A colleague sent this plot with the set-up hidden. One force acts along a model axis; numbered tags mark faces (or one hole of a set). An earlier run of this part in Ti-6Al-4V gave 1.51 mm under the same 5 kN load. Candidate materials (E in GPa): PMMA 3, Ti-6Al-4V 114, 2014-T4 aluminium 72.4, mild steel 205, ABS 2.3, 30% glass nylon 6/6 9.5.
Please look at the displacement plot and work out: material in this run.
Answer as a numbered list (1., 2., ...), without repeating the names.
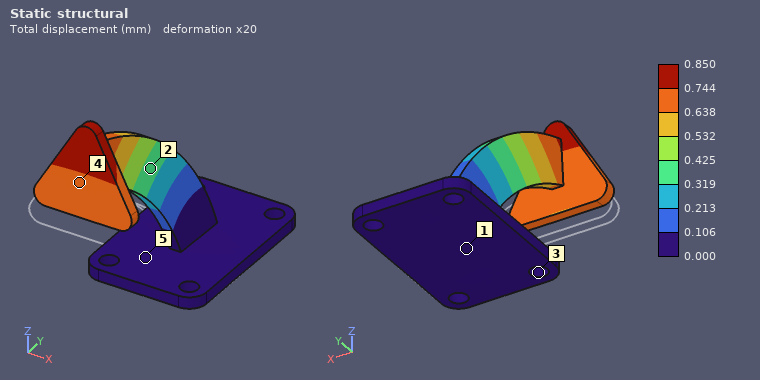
1. mild steel
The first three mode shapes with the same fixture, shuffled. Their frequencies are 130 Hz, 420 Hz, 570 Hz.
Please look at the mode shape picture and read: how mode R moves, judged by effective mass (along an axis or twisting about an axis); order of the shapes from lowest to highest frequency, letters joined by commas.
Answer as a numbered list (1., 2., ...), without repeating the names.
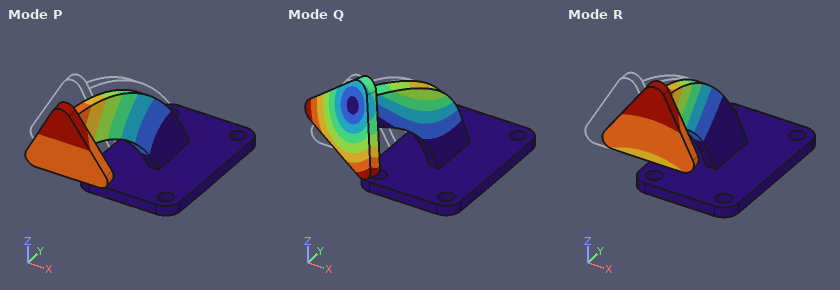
1. along X
2. R, P, Q
